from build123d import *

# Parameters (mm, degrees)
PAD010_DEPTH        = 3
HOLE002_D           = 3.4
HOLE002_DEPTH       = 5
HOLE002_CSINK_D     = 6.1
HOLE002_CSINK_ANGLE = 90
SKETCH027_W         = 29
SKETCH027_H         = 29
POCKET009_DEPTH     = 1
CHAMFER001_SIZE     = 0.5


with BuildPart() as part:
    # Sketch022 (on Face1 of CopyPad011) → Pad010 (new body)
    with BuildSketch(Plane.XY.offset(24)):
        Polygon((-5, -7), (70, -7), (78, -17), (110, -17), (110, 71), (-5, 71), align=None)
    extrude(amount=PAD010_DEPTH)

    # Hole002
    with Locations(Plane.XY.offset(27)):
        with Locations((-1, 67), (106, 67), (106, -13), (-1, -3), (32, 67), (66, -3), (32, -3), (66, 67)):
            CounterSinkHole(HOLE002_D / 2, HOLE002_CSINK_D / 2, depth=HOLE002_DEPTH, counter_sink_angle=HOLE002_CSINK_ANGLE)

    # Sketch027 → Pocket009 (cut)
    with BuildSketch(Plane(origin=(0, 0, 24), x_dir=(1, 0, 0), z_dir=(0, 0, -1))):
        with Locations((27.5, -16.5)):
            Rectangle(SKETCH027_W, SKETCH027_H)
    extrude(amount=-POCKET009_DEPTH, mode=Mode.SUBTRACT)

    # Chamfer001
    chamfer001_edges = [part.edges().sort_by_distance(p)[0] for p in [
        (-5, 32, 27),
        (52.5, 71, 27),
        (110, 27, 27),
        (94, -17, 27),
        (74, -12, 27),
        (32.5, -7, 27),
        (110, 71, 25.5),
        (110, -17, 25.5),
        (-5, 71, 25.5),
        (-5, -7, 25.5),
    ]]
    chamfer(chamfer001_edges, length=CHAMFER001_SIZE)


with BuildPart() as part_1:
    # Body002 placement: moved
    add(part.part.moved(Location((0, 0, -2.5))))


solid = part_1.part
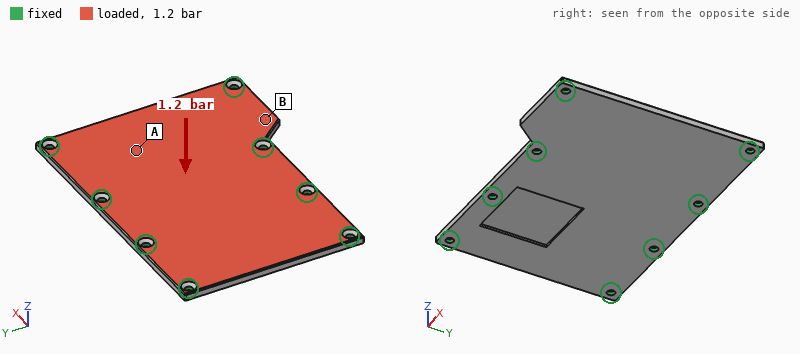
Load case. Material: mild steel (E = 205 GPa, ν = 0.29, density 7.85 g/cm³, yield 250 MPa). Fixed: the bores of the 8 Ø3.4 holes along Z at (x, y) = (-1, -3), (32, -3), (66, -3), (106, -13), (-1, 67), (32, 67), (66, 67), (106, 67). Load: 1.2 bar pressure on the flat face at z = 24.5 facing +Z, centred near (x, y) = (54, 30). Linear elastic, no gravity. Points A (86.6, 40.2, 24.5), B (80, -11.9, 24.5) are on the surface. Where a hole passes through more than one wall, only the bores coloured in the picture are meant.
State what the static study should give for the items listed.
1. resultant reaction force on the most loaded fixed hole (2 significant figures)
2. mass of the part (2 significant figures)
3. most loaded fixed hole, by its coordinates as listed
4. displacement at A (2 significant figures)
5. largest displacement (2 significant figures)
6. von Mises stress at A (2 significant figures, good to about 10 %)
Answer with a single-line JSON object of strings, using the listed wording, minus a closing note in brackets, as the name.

{"resultant reaction force on the most loaded fixed hole": "280 N", "mass of the part": "210 g", "most loaded fixed hole, by its coordinates as listed": "(66, -3)", "displacement at A": "30 µm", "largest displacement": "40 µm", "von Mises stress at A": "19 MPa"}
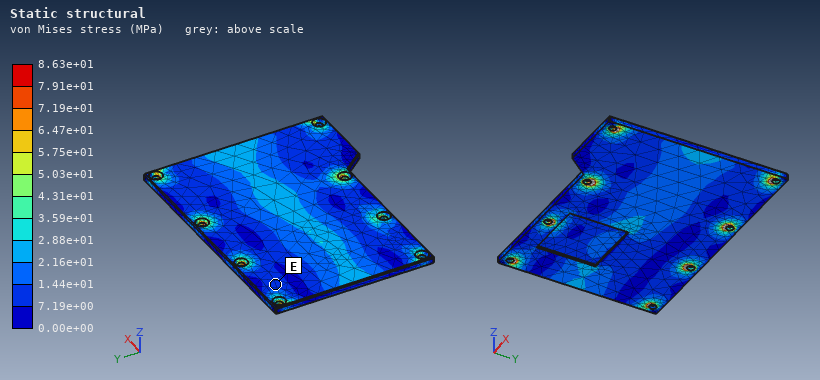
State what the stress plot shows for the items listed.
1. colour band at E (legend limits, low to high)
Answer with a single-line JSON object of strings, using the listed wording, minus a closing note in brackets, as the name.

{"colour band at E": "7.19e+00 to 1.44e+01 MPa"}
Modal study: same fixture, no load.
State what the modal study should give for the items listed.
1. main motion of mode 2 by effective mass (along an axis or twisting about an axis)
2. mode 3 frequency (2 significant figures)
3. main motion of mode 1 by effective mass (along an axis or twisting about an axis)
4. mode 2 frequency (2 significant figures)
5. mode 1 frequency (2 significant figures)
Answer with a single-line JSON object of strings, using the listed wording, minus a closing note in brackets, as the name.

{"main motion of mode 2 by effective mass": "along Z", "mode 3 frequency": "3700 Hz", "main motion of mode 1 by effective mass": "along Z", "mode 2 frequency": "2700 Hz", "mode 1 frequency": "2200 Hz"}
